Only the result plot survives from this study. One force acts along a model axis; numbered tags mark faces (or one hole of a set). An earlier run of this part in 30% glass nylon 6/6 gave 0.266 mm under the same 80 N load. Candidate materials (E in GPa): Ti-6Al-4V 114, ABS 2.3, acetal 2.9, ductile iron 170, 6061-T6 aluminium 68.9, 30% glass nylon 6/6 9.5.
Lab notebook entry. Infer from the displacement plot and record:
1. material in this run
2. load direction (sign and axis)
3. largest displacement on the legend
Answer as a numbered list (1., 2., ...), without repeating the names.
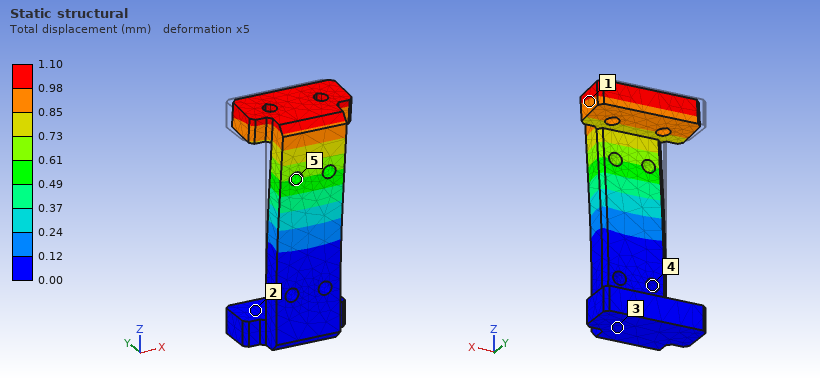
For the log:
1. ABS
2. -Y
3. 1.10 mm
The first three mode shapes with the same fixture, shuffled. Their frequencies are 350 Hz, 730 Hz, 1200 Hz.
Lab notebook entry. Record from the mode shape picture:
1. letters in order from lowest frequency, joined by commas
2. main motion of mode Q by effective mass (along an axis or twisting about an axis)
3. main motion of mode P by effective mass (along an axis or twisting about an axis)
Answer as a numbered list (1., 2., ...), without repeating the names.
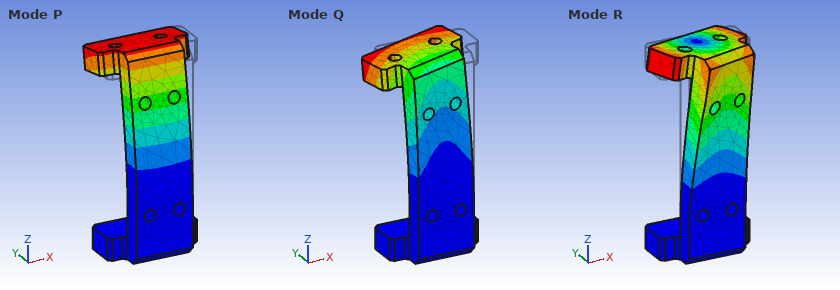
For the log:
1. P, Q, R
2. along X
3. along Y
